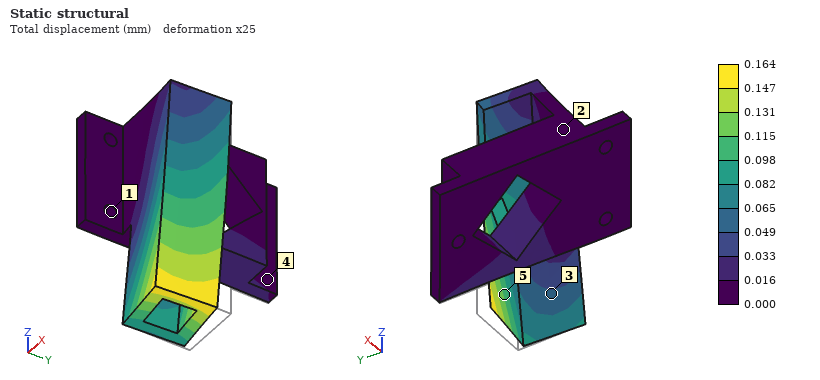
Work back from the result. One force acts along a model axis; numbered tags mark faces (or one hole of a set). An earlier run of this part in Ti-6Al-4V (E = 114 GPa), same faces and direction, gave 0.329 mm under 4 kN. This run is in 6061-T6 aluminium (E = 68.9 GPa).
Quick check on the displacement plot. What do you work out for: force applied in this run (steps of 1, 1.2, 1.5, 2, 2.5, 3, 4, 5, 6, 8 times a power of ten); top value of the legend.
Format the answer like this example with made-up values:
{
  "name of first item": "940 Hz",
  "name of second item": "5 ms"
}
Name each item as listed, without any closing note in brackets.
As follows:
{
  "force applied in this run": "1.2 kN",
  "top value of the legend": "0.164 mm"
}
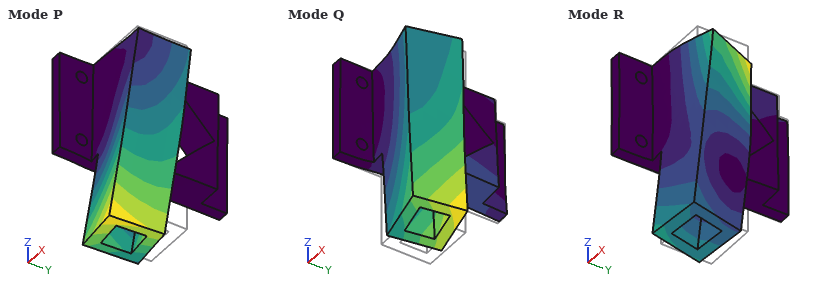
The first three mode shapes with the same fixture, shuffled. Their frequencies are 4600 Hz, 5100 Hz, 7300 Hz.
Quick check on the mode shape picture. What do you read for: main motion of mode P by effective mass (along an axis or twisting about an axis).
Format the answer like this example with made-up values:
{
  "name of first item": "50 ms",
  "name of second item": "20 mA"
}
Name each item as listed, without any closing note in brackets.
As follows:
{
  "main motion of mode P by effective mass": "along Y"
}
